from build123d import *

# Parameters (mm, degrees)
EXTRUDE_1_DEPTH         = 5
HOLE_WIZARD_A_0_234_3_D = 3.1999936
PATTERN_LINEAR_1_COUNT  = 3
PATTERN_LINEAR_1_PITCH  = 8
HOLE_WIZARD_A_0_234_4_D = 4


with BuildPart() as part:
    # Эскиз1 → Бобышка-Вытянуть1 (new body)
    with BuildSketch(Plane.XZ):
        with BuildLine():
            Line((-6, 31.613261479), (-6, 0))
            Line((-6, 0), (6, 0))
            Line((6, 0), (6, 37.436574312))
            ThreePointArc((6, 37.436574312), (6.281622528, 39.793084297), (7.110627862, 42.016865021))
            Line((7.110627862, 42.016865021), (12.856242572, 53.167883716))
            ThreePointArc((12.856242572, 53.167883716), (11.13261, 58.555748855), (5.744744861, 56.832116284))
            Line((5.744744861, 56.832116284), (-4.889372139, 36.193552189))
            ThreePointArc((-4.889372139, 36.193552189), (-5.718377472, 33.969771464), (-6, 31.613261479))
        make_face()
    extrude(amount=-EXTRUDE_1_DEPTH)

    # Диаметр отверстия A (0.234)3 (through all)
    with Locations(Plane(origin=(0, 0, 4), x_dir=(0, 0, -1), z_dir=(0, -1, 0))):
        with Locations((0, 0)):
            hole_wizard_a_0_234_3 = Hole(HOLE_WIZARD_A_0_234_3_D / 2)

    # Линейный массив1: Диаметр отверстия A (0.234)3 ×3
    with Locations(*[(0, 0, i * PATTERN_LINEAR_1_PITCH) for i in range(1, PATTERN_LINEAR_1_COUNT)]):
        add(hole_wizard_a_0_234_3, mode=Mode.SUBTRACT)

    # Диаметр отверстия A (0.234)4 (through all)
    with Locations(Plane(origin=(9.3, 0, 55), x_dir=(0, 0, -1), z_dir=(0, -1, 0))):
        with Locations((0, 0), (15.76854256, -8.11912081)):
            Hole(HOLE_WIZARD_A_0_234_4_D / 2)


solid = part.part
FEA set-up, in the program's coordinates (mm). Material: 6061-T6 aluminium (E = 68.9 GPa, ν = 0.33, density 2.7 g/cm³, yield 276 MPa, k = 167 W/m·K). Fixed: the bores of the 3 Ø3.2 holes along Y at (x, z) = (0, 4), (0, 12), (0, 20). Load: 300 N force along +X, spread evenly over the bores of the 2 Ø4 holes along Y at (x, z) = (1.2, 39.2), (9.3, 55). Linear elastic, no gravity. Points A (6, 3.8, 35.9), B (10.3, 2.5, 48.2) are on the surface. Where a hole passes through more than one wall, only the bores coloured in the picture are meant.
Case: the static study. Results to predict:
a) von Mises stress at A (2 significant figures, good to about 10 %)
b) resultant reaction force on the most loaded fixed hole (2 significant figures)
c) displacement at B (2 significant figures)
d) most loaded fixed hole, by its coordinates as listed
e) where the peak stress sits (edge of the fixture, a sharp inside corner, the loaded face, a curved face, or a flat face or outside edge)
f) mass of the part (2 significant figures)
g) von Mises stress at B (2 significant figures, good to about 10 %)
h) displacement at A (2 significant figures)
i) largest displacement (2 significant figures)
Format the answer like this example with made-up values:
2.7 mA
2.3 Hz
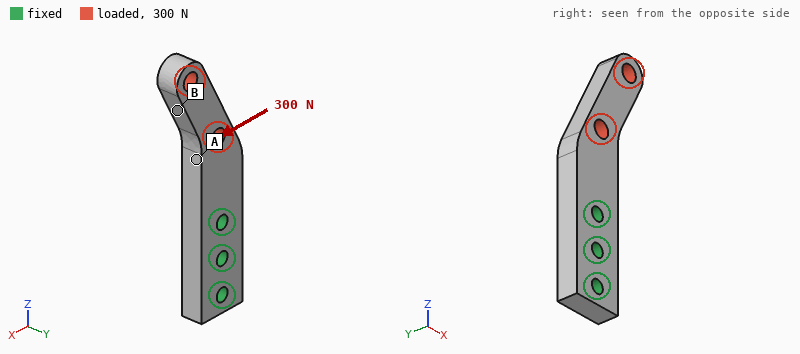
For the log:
42 MPa
770 N
0.083 mm
(0, 20)
edge of the fixture
7.9 g
13 MPa
0.034 mm
0.13 mm
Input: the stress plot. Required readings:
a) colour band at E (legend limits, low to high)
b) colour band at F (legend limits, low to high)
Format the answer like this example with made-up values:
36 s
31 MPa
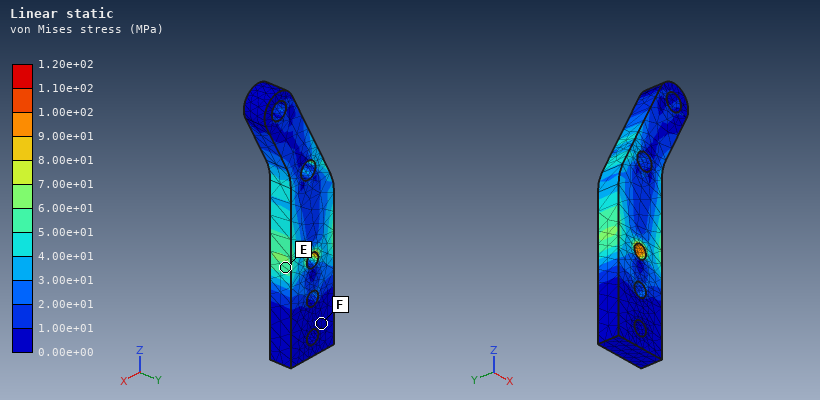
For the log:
5.00e+01 to 6.00e+01 MPa
0.00e+00 to 1.00e+01 MPa
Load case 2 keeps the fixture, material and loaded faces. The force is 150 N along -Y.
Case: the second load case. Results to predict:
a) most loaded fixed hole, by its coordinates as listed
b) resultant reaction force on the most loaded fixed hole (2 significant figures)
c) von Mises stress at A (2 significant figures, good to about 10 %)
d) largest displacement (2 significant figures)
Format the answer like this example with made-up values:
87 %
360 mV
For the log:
(0, 20)
270 N
31 MPa
0.25 mm
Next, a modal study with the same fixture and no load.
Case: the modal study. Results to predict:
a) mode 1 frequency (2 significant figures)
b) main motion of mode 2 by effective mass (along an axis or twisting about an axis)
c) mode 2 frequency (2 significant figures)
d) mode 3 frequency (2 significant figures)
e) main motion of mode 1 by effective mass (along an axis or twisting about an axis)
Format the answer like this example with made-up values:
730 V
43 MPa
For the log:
3200 Hz
along X
6100 Hz
14 kHz
along Y
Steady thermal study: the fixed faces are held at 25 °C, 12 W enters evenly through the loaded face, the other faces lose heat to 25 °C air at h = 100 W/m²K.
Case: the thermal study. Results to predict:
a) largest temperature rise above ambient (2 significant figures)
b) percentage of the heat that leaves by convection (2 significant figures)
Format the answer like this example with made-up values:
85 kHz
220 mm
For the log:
38 K
19 %
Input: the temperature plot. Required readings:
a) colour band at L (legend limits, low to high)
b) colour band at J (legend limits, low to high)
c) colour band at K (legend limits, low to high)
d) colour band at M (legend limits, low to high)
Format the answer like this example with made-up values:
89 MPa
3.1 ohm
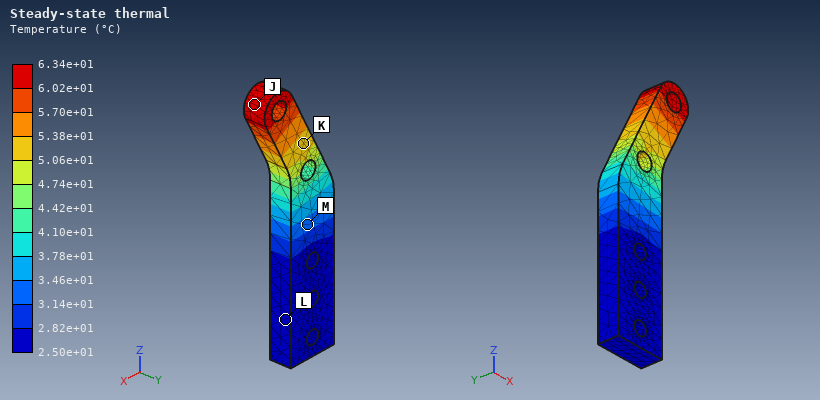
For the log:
2.50e+01 to 2.82e+01 °C
6.02e+01 to 6.34e+01 °C
5.06e+01 to 5.38e+01 °C
3.14e+01 to 3.46e+01 °C
